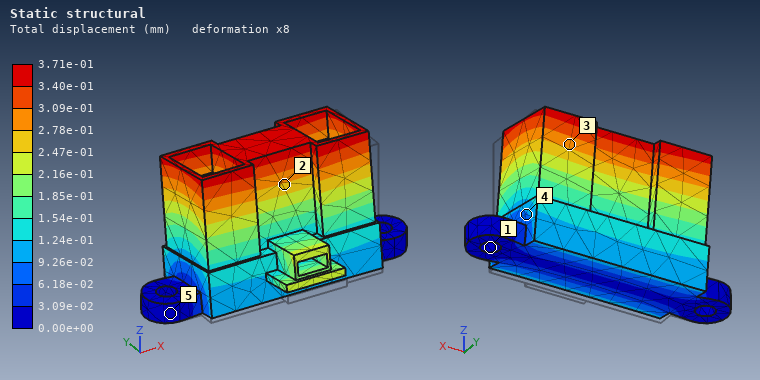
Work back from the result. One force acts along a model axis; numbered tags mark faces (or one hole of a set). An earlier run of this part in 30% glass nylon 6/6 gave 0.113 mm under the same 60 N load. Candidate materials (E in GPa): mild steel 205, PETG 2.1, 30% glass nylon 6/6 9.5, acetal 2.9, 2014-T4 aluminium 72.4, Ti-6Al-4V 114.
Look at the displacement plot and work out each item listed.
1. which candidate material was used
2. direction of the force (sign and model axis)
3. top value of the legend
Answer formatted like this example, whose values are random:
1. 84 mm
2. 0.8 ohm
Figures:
1. acetal
2. +Y
3. 3.71e-01 mm
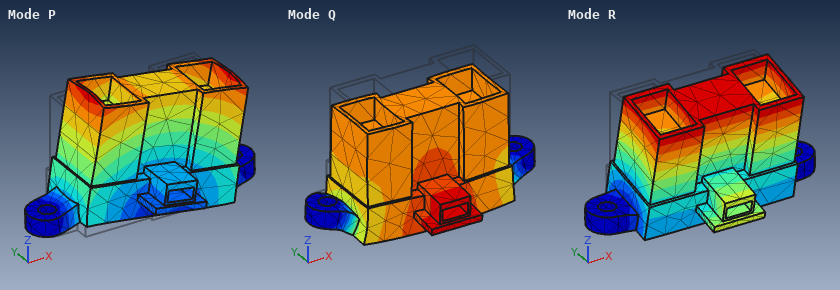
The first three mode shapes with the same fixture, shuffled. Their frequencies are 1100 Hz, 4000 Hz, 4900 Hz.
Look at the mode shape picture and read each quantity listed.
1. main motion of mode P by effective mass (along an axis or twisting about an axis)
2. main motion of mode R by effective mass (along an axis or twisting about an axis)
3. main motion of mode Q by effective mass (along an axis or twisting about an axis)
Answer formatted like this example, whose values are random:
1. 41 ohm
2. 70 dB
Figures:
1. along X
2. along Y
3. along Z
